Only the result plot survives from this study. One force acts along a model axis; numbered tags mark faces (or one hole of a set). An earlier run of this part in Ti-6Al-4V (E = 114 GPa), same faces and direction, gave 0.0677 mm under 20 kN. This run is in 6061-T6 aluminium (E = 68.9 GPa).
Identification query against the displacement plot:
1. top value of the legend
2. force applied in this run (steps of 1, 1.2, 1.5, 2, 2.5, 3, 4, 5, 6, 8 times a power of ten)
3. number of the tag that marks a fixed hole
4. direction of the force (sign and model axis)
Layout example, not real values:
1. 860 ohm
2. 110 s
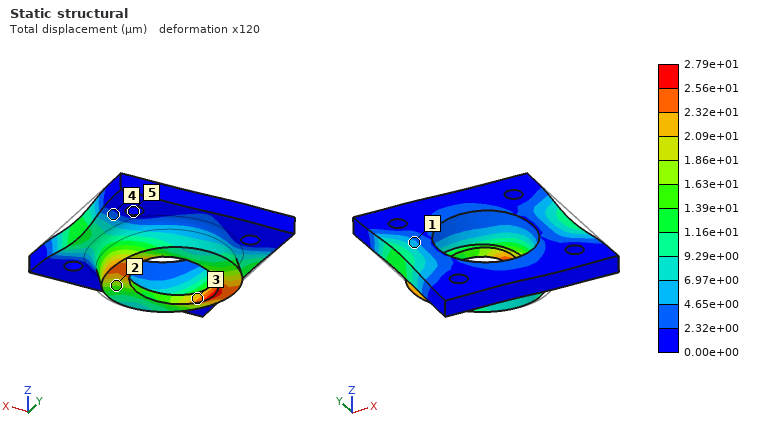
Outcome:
1. 2.79e+01 µm
2. 5 kN
3. 5
4. -X
